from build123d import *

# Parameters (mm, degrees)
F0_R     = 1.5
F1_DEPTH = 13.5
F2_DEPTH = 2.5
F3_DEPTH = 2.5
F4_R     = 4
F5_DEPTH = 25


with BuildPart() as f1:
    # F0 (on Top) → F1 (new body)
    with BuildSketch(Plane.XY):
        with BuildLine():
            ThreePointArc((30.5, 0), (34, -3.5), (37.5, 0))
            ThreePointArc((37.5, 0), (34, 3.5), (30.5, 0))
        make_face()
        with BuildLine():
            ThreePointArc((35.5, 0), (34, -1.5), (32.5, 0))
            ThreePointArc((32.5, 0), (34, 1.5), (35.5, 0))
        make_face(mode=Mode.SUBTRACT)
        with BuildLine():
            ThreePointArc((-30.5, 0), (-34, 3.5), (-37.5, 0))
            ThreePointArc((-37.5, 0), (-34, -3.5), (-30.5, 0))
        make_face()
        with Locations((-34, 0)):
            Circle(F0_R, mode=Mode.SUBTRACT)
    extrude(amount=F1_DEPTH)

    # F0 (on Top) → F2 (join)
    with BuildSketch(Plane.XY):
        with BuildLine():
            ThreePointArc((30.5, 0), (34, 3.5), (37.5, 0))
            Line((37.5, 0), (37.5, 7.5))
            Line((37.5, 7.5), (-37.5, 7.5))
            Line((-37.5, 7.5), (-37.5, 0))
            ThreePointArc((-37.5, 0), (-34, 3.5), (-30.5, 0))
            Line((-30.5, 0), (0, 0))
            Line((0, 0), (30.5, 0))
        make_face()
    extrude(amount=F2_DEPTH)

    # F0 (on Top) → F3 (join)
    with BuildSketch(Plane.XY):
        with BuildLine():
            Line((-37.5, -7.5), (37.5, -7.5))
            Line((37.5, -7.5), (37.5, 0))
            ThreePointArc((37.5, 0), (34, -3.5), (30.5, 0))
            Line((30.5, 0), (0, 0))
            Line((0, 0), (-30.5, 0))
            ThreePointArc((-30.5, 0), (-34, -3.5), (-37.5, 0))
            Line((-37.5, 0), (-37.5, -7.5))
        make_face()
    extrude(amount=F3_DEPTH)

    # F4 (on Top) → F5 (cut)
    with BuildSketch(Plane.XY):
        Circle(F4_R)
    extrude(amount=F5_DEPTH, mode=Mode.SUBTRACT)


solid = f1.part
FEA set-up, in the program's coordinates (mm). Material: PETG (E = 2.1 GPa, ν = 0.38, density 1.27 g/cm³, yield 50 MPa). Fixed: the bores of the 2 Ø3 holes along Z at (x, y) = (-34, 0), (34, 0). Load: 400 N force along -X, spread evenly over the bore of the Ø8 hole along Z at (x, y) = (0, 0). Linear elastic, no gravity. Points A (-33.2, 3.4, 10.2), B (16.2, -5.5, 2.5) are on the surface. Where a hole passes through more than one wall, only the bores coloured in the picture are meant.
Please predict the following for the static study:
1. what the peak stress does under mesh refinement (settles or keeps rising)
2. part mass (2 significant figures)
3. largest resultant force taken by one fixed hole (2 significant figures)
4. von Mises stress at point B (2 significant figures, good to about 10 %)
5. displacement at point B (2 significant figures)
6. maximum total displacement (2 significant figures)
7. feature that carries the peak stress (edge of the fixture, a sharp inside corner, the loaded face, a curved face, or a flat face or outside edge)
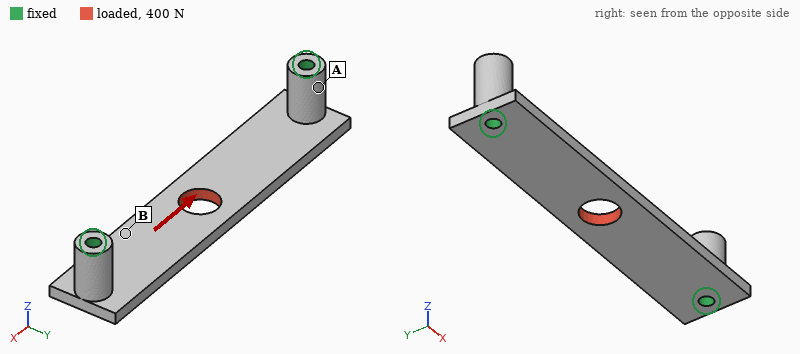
keeps rising
4.2 g
200 N
5.6 MPa
57 µm
99 µm
edge of the fixture
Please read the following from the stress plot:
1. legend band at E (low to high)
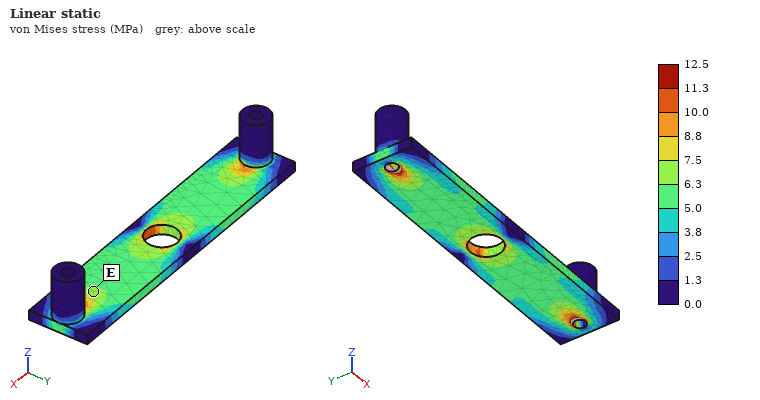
6.3 to 7.5 MPa
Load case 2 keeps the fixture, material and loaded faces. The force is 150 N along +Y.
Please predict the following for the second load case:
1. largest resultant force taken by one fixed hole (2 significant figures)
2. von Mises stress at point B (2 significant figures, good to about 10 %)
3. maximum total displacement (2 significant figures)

75 N
4.3 MPa
0.42 mm
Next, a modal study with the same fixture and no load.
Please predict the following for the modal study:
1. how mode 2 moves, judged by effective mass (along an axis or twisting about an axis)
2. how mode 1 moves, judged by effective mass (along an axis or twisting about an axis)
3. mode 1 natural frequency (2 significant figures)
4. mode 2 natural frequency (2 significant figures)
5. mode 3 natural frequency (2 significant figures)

twisting about X
along Z
780 Hz
2000 Hz
2100 Hz
